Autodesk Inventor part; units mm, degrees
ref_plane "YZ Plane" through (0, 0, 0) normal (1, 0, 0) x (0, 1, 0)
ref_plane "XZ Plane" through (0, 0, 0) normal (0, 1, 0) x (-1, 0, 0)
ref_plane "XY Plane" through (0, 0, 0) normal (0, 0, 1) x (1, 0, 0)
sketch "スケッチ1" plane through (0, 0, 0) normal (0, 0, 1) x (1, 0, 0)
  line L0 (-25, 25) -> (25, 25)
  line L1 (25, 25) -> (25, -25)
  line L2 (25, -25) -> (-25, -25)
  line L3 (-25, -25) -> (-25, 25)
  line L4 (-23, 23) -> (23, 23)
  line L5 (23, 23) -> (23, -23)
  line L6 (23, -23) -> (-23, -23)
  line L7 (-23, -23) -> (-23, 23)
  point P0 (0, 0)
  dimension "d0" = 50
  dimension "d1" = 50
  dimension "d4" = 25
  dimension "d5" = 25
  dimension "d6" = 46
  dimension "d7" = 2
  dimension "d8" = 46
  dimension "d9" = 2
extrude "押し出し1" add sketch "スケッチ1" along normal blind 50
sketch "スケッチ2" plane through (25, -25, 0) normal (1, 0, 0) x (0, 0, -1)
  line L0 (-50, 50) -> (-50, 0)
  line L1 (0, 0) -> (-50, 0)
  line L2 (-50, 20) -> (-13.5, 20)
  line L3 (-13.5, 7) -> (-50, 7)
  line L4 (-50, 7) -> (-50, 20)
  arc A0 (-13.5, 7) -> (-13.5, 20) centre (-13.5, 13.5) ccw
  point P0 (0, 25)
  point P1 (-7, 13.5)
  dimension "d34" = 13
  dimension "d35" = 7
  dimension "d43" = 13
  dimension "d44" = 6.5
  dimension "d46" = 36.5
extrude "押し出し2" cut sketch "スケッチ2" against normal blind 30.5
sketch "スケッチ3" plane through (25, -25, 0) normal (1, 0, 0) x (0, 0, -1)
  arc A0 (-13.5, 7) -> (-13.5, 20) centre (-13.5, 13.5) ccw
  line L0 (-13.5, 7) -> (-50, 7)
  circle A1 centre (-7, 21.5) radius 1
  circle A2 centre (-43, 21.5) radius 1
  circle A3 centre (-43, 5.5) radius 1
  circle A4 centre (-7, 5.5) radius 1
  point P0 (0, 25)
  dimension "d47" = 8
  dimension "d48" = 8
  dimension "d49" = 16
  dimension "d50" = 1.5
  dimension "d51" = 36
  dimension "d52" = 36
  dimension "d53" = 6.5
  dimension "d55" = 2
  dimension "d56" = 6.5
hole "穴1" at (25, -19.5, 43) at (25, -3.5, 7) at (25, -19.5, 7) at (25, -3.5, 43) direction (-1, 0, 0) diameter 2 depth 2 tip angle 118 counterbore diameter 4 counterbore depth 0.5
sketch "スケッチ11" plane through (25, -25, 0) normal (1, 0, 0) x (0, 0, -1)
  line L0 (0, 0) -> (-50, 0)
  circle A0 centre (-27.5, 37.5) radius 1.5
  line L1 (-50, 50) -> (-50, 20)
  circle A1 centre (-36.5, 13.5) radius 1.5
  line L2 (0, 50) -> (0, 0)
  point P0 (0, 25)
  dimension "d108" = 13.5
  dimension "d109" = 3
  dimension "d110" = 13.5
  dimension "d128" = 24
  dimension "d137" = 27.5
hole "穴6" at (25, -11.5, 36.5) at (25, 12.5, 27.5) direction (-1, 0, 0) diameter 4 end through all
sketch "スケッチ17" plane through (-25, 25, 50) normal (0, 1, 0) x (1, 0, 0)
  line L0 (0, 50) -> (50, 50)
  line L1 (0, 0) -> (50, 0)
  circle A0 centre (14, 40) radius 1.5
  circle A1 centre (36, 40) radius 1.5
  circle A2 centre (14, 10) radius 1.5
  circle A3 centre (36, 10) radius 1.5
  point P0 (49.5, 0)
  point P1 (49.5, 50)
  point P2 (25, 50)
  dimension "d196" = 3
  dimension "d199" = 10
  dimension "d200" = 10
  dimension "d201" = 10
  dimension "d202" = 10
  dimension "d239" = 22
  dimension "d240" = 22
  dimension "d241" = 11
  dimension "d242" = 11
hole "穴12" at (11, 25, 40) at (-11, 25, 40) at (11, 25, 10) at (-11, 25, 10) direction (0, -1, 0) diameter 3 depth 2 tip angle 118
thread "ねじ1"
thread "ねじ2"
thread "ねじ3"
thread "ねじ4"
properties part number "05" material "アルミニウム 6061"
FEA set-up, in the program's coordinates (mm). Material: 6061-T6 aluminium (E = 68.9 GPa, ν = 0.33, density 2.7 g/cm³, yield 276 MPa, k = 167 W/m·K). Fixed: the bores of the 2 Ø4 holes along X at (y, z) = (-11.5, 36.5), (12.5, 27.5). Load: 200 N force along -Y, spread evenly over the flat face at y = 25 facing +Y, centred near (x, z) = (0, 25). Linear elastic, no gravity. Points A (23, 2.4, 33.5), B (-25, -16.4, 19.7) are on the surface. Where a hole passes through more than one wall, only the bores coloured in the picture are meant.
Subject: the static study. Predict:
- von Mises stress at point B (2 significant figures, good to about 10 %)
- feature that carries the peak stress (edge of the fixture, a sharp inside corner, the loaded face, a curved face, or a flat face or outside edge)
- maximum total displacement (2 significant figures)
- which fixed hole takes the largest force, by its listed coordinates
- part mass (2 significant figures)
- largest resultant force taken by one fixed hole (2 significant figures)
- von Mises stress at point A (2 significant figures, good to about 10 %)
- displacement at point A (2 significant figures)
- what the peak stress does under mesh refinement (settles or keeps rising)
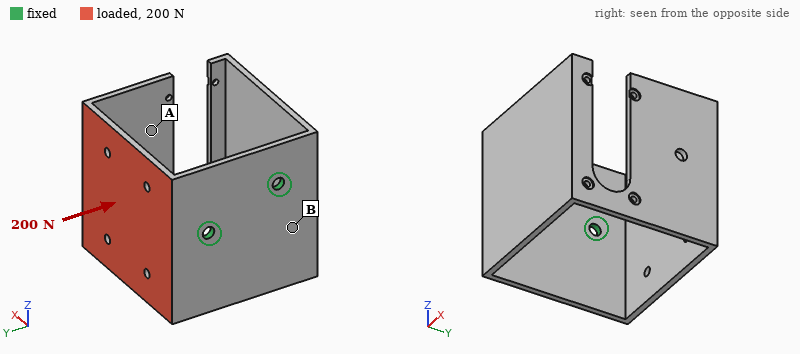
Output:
30 MPa
edge of the fixture
0.94 mm
(12.5, 27.5)
48 g
170 N
14 MPa
0.83 mm
keeps rising
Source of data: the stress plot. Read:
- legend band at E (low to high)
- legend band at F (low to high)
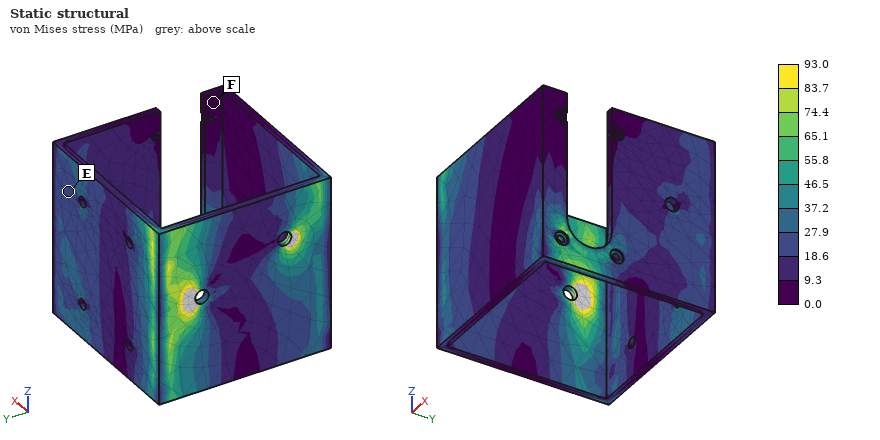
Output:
18.6 to 27.9 MPa
0.0 to 9.3 MPa
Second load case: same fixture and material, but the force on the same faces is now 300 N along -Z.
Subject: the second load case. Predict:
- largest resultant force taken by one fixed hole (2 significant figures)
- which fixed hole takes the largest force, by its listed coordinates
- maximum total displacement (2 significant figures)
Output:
410 N
(12.5, 27.5)
0.90 mm
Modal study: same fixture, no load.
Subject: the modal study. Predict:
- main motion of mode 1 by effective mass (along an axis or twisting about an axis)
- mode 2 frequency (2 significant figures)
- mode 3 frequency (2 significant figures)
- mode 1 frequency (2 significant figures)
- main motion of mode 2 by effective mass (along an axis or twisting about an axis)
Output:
along Y
530 Hz
980 Hz
400 Hz
along Z
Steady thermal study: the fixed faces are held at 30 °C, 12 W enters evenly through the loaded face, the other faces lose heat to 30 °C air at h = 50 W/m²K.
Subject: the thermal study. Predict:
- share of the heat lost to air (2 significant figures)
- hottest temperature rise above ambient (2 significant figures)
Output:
43 %
16 K
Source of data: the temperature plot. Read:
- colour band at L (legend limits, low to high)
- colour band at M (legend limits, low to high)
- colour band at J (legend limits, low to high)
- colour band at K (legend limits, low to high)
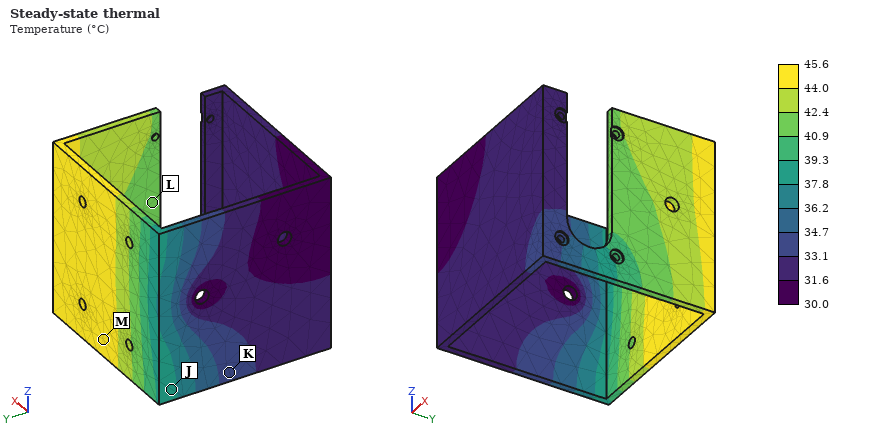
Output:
40.9 to 42.4 °C
44.0 to 45.6 °C
37.8 to 39.3 °C
33.1 to 34.7 °C
